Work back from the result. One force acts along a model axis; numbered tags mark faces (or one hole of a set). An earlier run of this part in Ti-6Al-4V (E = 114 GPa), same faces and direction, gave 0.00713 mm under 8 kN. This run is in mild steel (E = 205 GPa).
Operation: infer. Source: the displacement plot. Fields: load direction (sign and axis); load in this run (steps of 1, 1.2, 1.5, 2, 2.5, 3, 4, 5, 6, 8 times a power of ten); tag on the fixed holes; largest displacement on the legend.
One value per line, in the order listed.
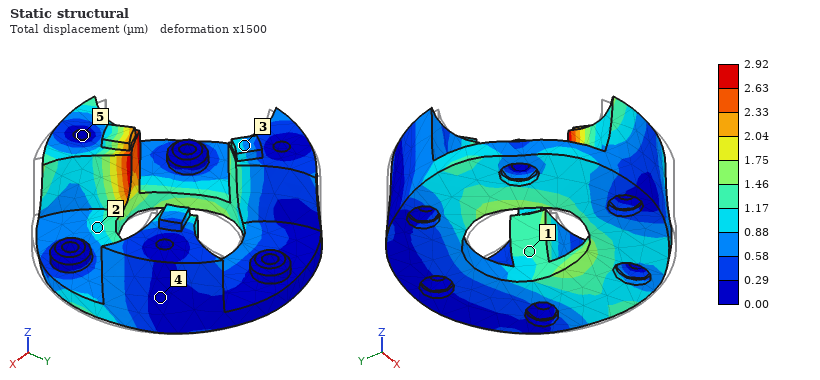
-X
6 kN
5
2.92 µm
